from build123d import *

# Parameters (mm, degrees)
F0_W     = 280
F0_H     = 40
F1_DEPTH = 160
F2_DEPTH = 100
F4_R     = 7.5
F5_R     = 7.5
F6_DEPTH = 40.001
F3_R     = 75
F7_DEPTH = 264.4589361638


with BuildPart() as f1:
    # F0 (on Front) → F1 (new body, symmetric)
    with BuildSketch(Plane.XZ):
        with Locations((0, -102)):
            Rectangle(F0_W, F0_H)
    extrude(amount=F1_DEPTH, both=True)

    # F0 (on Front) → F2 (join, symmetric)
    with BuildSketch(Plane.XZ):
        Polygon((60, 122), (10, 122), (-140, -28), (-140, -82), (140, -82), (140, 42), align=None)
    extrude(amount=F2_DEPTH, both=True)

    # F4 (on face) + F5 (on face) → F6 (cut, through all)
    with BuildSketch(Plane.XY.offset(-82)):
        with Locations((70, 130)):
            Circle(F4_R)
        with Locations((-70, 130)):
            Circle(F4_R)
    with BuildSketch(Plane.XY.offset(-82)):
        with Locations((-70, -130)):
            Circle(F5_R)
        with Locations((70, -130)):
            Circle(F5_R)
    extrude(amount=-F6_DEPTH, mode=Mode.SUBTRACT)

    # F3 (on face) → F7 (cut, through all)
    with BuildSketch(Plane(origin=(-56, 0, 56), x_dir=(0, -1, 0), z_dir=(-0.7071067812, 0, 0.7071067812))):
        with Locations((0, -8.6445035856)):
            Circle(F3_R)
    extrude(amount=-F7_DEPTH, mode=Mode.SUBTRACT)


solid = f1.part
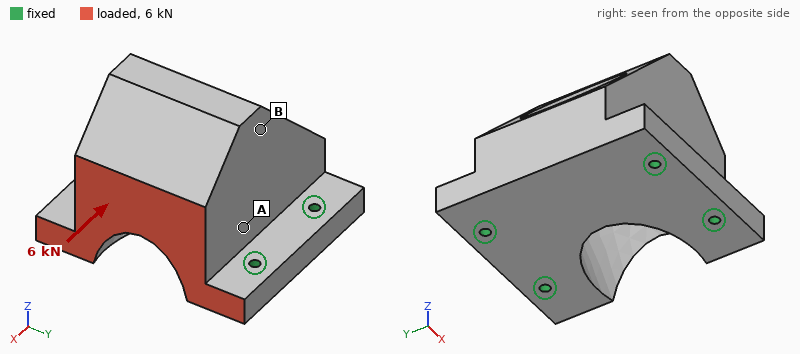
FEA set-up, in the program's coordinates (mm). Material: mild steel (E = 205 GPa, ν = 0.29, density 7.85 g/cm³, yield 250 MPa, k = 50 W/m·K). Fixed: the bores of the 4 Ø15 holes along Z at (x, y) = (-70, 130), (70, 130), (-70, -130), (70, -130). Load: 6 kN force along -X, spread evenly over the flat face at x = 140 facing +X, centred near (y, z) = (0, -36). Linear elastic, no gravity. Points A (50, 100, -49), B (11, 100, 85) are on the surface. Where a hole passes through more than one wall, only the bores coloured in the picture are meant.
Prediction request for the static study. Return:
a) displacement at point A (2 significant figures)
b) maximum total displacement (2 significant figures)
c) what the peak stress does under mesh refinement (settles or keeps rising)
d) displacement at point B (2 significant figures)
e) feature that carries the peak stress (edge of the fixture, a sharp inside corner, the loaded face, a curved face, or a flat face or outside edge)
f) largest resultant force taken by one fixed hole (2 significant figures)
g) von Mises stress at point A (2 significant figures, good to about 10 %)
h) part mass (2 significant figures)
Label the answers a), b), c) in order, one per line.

a) 0.88 µm
b) 2.3 µm
c) keeps rising
d) 1.9 µm
e) edge of the fixture
f) 2.2 kN
g) 0.80 MPa
h) 63 kg
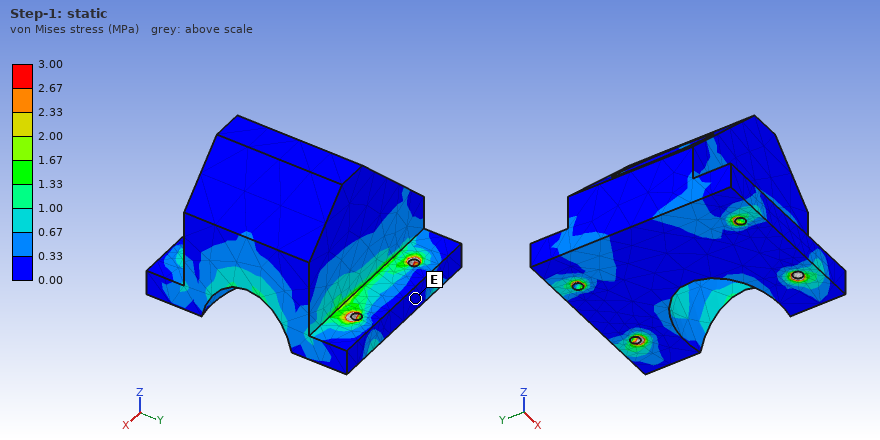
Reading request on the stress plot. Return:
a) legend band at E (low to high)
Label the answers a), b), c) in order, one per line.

a) 0.00 to 0.33 MPa
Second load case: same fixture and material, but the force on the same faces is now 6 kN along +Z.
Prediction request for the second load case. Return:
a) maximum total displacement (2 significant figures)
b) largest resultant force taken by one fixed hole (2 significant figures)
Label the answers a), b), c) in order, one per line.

a) 3.6 µm
b) 4.2 kN
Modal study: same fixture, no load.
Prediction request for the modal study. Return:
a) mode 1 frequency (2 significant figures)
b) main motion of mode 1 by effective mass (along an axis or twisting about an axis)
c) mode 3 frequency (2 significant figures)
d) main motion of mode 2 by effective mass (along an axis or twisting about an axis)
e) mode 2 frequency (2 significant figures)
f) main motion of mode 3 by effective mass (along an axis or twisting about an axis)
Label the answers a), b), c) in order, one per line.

a) 1100 Hz
b) along X
c) 2100 Hz
d) along Y
e) 1400 Hz
f) along Z
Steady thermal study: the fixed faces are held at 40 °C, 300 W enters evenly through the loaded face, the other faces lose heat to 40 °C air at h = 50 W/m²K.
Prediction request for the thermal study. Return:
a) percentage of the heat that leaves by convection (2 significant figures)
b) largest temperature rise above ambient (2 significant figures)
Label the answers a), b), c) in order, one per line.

a) 60 %
b) 38 K
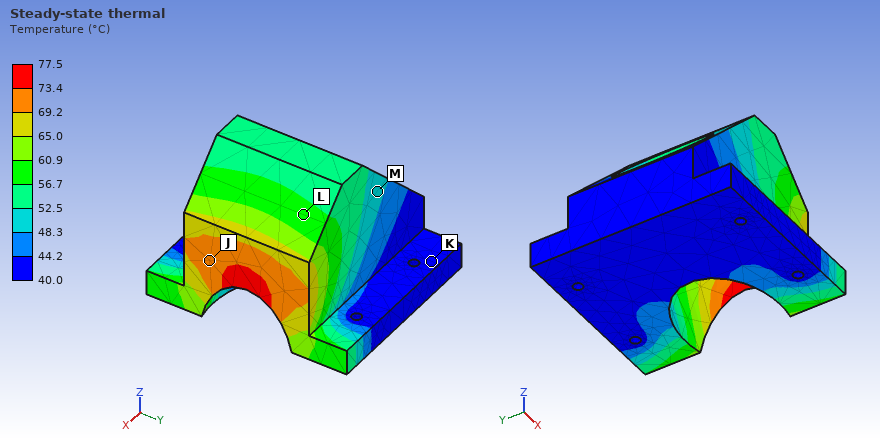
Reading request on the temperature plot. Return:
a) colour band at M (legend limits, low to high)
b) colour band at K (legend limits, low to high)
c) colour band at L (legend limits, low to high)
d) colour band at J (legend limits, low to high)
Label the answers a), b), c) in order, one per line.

a) 48.3 to 52.5 °C
b) 40.0 to 44.2 °C
c) 56.7 to 60.9 °C
d) 69.2 to 73.4 °C
